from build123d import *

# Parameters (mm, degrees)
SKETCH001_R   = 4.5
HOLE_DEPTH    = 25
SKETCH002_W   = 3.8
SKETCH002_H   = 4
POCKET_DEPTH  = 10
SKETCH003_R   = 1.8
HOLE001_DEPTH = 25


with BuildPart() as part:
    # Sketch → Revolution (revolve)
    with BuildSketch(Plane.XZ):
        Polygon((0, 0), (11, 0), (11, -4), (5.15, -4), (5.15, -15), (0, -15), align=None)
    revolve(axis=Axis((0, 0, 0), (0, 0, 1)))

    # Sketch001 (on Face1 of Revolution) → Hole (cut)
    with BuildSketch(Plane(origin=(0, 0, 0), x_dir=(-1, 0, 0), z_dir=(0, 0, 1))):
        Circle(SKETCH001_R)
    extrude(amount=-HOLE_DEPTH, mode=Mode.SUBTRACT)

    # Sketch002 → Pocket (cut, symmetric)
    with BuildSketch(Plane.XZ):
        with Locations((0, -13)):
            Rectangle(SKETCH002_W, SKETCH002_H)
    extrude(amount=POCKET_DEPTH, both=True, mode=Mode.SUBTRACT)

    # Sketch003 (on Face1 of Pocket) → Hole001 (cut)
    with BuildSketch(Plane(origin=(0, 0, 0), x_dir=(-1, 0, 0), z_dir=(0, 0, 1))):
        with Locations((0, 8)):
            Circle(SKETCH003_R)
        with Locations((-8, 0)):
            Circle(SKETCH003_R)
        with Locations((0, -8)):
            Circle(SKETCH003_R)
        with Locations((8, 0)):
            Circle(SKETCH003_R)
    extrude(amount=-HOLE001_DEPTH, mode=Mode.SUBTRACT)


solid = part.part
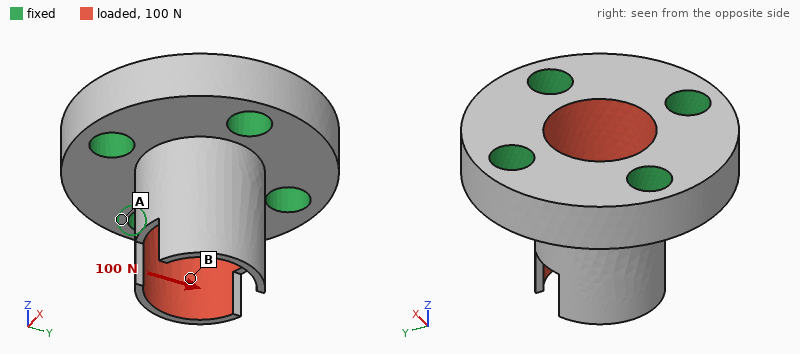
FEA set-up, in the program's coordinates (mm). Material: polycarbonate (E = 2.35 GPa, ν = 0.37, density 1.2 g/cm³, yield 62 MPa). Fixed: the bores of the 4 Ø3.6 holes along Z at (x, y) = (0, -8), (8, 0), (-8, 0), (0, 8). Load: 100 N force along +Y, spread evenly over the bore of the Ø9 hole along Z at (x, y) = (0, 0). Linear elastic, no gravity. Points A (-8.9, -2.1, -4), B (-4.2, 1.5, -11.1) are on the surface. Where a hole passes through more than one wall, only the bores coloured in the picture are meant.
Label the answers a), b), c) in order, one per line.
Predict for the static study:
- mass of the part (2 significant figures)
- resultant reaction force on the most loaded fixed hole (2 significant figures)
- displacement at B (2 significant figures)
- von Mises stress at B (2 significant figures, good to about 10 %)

a) 1.6 g
b) 44 N
c) 0.076 mm
d) 8.1 MPa
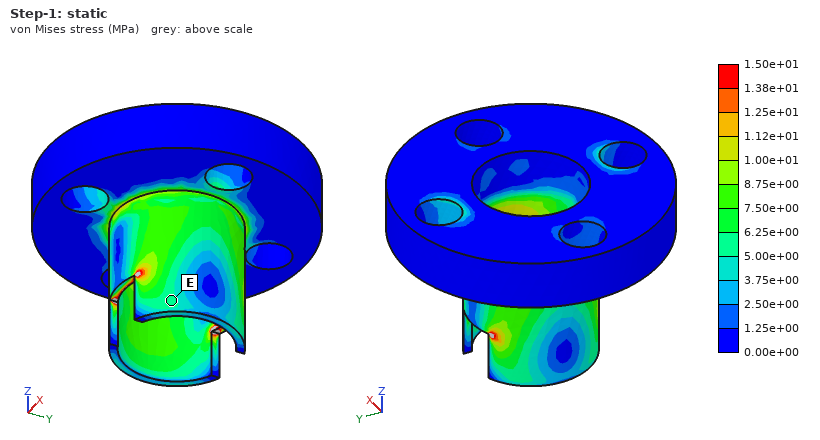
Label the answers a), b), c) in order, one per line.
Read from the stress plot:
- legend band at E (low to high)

a) 5.00e+00 to 6.25e+00 MPa
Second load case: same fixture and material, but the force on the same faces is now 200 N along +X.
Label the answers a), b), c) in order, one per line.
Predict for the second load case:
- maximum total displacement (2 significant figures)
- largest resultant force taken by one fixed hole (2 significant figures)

a) 0.25 mm
b) 88 N
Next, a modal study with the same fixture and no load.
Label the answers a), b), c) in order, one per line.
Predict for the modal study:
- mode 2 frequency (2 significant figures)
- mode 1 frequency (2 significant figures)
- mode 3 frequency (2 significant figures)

a) 7600 Hz
b) 6100 Hz
c) 7800 Hz
